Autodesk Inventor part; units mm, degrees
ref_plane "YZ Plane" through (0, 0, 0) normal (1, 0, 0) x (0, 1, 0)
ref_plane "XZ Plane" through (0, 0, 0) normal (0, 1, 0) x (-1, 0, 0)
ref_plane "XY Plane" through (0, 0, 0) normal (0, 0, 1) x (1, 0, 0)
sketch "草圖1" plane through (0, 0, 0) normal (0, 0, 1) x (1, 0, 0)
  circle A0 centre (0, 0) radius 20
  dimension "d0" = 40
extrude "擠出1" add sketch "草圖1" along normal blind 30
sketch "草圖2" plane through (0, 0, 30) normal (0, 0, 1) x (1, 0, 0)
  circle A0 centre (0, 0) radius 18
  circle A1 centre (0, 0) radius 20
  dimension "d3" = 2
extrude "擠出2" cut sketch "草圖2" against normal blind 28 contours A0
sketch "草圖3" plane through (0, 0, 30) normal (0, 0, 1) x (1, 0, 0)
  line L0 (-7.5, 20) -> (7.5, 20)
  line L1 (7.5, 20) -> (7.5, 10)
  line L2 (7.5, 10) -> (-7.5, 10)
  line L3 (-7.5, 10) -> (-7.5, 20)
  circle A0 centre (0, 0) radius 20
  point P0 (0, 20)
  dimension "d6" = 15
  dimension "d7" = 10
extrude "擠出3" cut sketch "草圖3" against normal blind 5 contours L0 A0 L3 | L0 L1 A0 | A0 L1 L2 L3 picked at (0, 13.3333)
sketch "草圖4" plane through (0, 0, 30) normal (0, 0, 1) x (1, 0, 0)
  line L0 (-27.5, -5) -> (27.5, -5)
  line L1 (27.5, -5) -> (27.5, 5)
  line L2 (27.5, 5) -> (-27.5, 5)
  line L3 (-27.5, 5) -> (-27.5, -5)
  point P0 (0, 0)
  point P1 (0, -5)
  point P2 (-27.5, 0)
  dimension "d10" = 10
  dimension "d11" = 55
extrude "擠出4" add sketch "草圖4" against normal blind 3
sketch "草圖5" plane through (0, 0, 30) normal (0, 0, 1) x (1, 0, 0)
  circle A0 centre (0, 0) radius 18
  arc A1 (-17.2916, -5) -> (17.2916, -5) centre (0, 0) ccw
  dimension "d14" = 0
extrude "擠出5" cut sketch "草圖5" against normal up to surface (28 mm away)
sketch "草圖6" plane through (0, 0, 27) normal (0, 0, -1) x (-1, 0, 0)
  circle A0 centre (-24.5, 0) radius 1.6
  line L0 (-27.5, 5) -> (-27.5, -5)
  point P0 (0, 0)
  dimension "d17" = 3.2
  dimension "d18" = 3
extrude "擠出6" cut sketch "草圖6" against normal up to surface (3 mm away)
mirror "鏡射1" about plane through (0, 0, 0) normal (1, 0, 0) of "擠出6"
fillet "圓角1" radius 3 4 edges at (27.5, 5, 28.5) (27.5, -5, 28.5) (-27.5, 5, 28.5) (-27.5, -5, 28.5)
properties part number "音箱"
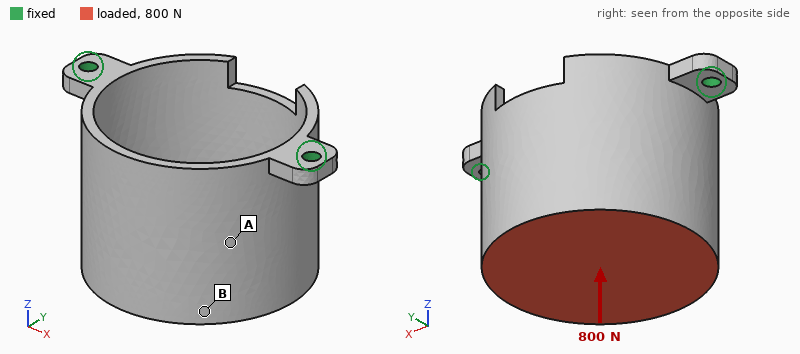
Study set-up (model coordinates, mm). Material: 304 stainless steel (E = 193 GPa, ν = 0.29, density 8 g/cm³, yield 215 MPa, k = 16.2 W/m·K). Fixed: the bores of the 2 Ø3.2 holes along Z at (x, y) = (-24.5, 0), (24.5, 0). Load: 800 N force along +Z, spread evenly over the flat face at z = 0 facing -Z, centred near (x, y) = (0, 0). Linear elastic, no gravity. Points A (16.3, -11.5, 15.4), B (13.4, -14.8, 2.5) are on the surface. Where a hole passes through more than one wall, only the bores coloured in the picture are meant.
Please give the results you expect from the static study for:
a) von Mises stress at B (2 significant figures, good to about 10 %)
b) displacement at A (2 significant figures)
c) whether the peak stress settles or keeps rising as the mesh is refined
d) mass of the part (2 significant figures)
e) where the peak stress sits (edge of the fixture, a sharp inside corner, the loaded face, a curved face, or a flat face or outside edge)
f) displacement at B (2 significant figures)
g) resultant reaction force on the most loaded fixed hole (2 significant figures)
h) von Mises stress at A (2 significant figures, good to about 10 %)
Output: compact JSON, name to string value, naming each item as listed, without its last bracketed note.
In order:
{"von Mises stress at B": "17 MPa", "displacement at A": "4.4 µm", "whether the peak stress settles or keeps rising as the mesh is refined": "keeps rising", "mass of the part": "75 g", "where the peak stress sits": "edge of the fixture", "displacement at B": "4.5 µm", "resultant reaction force on the most loaded fixed hole": "410 N", "von Mises stress at A": "6.4 MPa"}
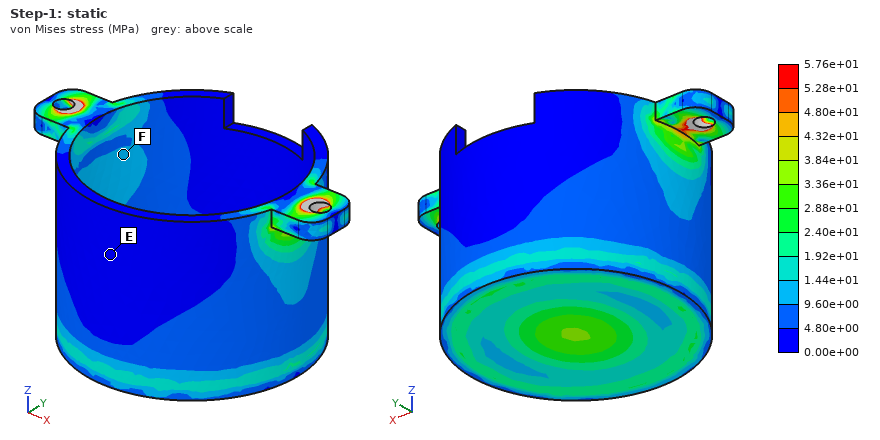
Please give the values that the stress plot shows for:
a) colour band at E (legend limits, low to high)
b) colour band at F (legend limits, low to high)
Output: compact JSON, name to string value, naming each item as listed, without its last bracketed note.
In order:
{"colour band at E": "0.00e+00 to 4.80e+00 MPa", "colour band at F": "9.60e+00 to 1.44e+01 MPa"}
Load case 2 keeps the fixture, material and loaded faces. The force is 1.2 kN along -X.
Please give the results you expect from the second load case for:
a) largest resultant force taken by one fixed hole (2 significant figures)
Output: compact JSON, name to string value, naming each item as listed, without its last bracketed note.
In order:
{"largest resultant force taken by one fixed hole": "1.0 kN"}
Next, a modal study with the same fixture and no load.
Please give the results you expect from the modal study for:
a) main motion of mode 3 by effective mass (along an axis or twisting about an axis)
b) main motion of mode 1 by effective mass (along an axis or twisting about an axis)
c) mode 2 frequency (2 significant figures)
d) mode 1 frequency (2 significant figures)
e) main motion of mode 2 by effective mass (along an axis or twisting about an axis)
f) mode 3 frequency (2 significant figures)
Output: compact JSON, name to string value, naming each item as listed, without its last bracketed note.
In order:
{"main motion of mode 3 by effective mass": "twisting about Z", "main motion of mode 1 by effective mass": "along Y", "mode 2 frequency": "4500 Hz", "mode 1 frequency": "1300 Hz", "main motion of mode 2 by effective mass": "along X", "mode 3 frequency": "5400 Hz"}
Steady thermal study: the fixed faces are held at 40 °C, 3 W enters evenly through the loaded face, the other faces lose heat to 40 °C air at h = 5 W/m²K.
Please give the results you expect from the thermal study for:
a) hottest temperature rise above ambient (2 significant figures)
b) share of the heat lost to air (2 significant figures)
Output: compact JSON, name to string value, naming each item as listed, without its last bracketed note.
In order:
{"hottest temperature rise above ambient": "41 K", "share of the heat lost to air": "37 %"}
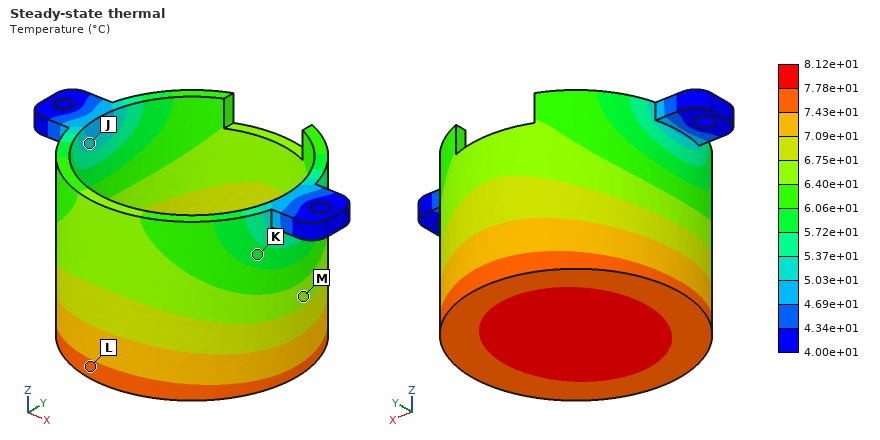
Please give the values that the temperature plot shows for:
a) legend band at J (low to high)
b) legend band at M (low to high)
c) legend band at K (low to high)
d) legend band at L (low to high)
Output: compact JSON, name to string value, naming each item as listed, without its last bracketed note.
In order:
{"legend band at J": "5.03e+01 to 5.37e+01 °C", "legend band at M": "6.40e+01 to 6.75e+01 °C", "legend band at K": "5.72e+01 to 6.06e+01 °C", "legend band at L": "7.43e+01 to 7.78e+01 °C"}
